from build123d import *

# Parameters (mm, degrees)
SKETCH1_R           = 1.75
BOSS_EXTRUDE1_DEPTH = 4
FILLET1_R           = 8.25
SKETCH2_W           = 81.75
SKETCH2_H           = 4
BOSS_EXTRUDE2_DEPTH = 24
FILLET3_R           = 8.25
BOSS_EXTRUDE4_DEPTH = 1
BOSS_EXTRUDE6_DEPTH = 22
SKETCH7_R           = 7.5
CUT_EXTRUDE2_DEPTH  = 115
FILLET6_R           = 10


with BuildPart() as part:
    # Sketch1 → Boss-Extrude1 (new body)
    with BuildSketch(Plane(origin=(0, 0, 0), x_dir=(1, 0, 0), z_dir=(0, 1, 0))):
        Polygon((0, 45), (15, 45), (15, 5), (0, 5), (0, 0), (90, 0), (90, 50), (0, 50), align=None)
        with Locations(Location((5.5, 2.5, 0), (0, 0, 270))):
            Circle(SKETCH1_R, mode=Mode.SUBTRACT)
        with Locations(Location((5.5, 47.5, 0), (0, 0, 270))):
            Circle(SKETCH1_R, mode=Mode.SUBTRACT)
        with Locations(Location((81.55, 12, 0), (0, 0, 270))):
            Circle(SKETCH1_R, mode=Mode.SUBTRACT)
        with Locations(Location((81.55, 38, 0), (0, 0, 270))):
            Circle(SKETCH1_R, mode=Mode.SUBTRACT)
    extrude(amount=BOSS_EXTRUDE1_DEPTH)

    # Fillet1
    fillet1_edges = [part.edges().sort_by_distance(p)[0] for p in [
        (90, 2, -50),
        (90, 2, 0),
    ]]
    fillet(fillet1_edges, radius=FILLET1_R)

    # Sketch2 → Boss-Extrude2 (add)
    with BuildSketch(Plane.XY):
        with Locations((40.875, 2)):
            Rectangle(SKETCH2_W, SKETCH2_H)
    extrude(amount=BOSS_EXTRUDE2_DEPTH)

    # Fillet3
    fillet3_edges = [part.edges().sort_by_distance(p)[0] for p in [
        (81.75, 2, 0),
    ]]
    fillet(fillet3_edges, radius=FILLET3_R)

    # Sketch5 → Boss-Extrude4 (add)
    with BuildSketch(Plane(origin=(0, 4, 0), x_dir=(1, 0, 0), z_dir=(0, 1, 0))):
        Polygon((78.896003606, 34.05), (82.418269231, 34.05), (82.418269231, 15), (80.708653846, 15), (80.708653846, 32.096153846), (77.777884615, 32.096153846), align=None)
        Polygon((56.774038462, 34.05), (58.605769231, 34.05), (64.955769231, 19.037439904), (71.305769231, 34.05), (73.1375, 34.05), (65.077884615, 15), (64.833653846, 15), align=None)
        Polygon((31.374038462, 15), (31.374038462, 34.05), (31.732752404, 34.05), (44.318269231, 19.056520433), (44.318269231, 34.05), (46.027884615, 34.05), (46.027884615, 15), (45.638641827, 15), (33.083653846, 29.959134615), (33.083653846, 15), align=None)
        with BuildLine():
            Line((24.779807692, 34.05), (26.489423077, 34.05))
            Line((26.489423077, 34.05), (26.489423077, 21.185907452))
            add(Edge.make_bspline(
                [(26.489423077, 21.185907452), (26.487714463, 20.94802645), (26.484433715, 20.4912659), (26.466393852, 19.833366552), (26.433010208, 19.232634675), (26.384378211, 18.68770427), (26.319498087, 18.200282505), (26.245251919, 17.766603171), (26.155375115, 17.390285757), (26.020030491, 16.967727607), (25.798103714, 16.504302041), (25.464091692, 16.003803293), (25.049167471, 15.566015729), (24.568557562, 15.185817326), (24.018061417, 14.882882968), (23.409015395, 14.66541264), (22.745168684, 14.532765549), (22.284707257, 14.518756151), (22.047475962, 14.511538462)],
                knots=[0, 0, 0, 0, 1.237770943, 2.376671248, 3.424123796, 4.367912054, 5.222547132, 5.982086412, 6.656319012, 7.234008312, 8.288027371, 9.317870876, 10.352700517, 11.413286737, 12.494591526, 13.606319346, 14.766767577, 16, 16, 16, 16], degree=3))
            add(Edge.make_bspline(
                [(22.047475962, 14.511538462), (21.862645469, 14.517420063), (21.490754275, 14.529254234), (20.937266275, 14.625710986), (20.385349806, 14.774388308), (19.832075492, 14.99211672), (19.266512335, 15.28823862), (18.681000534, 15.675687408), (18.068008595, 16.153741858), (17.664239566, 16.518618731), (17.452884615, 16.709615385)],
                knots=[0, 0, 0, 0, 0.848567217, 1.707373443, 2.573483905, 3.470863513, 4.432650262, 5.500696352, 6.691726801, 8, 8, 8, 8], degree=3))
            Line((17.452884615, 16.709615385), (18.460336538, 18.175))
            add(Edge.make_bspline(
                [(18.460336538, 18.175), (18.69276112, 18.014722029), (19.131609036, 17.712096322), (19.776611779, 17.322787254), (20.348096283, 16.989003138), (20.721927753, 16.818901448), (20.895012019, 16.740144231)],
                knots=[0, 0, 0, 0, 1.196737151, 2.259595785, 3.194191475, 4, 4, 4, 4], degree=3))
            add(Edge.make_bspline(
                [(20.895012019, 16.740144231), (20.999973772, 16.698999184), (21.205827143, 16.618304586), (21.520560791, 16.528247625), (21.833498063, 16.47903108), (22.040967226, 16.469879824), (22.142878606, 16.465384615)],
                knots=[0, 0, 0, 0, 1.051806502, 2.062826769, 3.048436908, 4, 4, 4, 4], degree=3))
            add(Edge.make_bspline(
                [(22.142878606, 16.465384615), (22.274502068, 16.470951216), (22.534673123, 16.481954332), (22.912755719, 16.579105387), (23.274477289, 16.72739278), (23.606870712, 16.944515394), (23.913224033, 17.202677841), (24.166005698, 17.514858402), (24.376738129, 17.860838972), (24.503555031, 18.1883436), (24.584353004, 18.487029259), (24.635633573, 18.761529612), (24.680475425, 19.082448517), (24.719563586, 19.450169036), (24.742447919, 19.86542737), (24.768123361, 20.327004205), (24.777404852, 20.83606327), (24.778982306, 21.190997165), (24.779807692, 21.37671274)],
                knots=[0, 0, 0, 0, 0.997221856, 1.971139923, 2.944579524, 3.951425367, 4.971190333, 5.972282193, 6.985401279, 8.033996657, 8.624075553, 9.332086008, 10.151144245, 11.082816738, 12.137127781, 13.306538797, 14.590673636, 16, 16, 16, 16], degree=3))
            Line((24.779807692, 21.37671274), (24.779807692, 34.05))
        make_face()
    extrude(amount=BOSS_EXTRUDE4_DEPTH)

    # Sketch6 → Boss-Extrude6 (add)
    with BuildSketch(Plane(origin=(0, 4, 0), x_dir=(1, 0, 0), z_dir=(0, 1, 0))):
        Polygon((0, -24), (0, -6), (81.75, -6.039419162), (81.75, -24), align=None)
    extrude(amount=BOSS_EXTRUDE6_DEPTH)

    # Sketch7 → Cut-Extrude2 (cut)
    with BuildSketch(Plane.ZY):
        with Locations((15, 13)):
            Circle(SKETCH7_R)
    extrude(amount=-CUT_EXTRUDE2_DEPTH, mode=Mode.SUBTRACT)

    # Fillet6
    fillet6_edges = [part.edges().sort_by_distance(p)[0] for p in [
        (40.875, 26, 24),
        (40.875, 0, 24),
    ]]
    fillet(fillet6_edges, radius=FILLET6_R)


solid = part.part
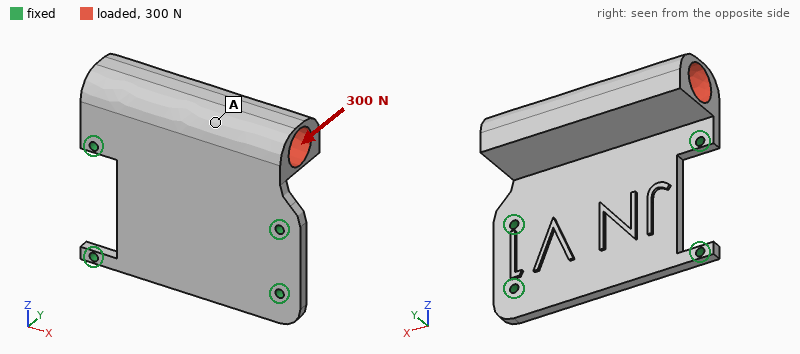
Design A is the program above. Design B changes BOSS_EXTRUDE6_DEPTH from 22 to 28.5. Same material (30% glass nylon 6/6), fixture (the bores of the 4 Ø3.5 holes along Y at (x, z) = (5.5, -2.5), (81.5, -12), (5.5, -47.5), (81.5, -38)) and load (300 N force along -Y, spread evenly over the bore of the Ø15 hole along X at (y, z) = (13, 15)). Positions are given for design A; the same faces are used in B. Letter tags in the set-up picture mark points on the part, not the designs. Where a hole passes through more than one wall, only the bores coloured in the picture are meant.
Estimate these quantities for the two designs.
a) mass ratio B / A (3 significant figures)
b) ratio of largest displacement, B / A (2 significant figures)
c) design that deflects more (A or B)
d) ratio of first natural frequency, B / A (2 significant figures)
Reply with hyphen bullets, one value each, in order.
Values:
- 1.25
- 1.1
- B
- 0.72
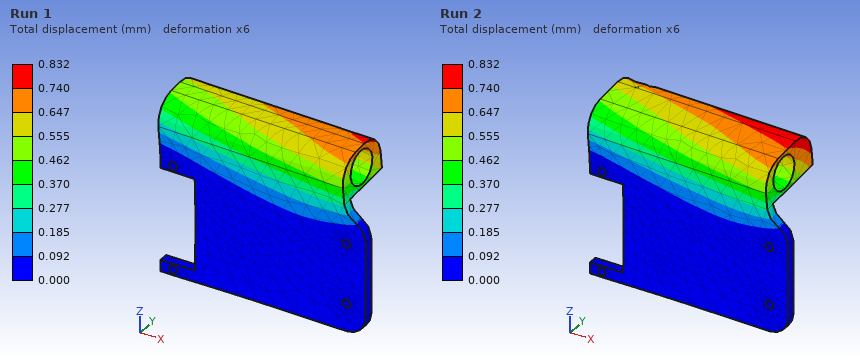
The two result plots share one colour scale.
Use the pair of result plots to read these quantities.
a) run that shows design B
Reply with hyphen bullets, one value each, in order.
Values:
- Run 2
